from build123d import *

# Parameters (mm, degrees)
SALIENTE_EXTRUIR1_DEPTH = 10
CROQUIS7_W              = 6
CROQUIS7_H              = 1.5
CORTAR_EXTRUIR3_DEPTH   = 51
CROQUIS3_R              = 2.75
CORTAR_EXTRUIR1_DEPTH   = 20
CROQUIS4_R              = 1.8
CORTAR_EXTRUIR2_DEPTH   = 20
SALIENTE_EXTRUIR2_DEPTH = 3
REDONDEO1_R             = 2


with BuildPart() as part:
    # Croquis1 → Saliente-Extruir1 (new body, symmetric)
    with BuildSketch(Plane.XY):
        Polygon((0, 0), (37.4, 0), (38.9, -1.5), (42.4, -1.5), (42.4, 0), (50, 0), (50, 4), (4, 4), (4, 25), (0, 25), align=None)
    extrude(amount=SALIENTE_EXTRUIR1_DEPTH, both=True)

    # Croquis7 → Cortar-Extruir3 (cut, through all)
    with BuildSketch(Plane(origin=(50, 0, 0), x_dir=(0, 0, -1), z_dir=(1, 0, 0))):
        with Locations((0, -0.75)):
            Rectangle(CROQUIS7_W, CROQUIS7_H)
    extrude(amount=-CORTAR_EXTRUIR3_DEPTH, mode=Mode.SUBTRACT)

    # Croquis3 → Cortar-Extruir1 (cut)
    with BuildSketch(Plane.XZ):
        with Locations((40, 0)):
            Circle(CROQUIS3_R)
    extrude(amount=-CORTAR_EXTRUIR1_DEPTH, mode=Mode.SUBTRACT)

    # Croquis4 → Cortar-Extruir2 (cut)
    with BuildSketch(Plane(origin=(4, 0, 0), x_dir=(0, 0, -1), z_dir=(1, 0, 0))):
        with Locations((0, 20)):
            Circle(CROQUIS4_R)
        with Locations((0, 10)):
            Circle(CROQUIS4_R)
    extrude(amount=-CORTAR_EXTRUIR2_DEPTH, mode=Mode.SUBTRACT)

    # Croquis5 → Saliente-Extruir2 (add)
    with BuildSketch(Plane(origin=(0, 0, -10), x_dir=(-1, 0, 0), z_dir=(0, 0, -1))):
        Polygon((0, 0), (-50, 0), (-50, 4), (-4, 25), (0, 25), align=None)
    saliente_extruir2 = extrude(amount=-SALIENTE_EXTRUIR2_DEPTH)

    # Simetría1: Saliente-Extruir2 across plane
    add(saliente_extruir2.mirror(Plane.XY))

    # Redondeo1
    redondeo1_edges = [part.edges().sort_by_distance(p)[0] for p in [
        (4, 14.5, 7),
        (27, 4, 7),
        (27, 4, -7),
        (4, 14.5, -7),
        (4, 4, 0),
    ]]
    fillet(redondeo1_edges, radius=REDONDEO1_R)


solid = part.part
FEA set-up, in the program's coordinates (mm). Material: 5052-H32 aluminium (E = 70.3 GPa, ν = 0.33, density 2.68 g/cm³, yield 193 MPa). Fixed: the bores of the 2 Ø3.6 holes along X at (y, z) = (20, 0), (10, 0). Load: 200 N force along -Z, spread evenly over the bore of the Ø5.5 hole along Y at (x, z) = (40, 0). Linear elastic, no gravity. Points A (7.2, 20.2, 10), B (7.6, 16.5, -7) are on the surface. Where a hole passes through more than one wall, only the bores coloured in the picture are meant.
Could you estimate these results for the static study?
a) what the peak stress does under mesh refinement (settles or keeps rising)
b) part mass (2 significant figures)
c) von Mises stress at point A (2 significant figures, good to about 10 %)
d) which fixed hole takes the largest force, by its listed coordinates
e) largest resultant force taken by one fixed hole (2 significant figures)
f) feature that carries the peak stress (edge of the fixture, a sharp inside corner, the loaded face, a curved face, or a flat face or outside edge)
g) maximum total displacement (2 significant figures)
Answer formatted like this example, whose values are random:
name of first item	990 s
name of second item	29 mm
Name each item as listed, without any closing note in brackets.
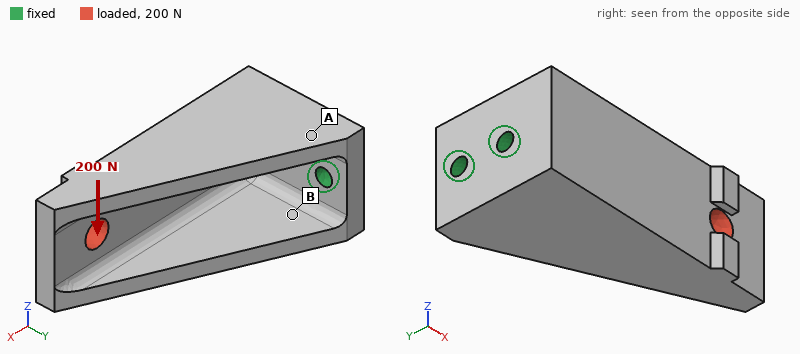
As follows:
what the peak stress does under mesh refinement	keeps rising
part mass	23 g
von Mises stress at point A	18 MPa
which fixed hole takes the largest force, by its listed coordinates	(10, 0)
largest resultant force taken by one fixed hole	290 N
feature that carries the peak stress	edge of the fixture
maximum total displacement	0.12 mm
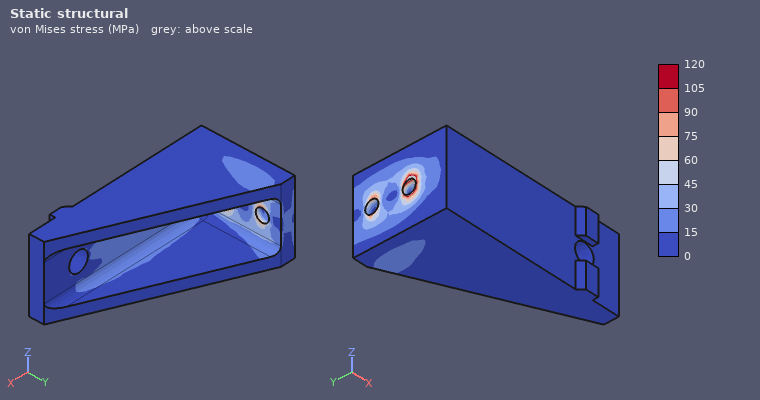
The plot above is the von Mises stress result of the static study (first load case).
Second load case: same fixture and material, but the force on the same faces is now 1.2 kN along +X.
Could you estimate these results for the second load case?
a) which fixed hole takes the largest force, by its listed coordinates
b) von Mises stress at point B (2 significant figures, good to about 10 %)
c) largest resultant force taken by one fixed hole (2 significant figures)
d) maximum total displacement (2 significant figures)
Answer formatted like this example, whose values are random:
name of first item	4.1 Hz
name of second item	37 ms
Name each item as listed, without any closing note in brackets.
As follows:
which fixed hole takes the largest force, by its listed coordinates	(10, 0)
von Mises stress at point B	10 MPa
largest resultant force taken by one fixed hole	1.6 kN
maximum total displacement	83 µm
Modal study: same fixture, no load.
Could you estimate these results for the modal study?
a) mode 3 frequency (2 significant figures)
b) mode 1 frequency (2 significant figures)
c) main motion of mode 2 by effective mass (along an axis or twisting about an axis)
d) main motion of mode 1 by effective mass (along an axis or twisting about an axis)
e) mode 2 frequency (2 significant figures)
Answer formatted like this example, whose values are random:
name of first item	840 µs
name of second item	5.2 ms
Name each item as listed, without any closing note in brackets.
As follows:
mode 3 frequency	9000 Hz
mode 1 frequency	2500 Hz
main motion of mode 2 by effective mass	along Y
main motion of mode 1 by effective mass	along Z
mode 2 frequency	3900 Hz
